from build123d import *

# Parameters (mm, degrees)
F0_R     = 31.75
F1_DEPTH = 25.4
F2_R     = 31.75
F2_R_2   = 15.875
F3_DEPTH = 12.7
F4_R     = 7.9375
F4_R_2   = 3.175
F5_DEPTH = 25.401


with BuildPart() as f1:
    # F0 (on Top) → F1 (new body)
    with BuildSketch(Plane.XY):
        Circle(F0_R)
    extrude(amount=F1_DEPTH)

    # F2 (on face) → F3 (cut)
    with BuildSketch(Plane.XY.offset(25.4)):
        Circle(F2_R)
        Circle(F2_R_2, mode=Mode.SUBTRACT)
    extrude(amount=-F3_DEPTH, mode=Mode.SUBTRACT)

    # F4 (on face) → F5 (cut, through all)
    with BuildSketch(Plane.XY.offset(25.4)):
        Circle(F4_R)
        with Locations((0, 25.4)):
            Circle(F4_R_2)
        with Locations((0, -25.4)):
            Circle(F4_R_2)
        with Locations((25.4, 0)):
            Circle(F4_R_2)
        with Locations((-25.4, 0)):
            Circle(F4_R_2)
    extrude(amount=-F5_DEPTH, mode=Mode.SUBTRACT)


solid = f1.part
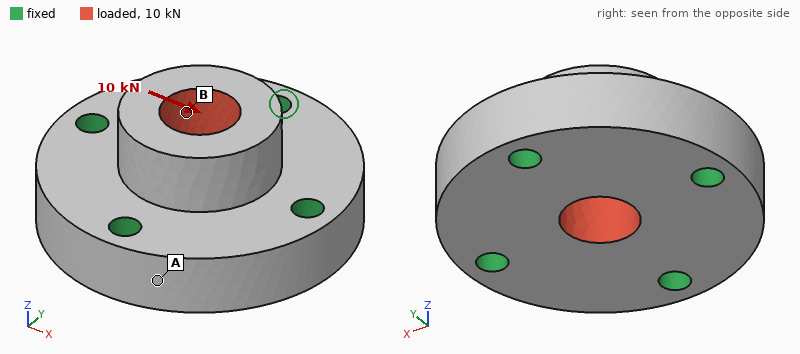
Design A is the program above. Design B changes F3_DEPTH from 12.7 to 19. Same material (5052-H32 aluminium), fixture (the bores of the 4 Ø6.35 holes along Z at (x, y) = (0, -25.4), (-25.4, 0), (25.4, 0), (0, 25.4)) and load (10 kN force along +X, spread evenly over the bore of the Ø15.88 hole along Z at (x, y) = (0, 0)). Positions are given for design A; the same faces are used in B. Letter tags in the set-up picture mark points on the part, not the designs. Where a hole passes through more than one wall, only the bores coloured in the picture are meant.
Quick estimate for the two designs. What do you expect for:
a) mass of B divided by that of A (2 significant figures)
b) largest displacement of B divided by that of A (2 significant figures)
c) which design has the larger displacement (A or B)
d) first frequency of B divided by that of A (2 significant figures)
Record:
0.68
3.1
B
0.59
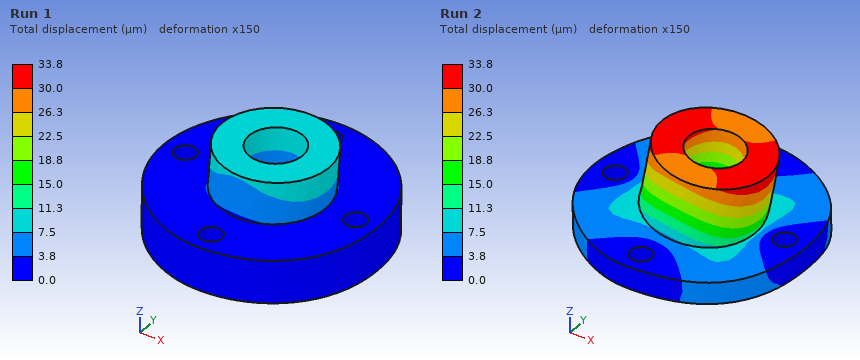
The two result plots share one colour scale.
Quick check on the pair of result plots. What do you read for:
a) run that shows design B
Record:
Run 2
